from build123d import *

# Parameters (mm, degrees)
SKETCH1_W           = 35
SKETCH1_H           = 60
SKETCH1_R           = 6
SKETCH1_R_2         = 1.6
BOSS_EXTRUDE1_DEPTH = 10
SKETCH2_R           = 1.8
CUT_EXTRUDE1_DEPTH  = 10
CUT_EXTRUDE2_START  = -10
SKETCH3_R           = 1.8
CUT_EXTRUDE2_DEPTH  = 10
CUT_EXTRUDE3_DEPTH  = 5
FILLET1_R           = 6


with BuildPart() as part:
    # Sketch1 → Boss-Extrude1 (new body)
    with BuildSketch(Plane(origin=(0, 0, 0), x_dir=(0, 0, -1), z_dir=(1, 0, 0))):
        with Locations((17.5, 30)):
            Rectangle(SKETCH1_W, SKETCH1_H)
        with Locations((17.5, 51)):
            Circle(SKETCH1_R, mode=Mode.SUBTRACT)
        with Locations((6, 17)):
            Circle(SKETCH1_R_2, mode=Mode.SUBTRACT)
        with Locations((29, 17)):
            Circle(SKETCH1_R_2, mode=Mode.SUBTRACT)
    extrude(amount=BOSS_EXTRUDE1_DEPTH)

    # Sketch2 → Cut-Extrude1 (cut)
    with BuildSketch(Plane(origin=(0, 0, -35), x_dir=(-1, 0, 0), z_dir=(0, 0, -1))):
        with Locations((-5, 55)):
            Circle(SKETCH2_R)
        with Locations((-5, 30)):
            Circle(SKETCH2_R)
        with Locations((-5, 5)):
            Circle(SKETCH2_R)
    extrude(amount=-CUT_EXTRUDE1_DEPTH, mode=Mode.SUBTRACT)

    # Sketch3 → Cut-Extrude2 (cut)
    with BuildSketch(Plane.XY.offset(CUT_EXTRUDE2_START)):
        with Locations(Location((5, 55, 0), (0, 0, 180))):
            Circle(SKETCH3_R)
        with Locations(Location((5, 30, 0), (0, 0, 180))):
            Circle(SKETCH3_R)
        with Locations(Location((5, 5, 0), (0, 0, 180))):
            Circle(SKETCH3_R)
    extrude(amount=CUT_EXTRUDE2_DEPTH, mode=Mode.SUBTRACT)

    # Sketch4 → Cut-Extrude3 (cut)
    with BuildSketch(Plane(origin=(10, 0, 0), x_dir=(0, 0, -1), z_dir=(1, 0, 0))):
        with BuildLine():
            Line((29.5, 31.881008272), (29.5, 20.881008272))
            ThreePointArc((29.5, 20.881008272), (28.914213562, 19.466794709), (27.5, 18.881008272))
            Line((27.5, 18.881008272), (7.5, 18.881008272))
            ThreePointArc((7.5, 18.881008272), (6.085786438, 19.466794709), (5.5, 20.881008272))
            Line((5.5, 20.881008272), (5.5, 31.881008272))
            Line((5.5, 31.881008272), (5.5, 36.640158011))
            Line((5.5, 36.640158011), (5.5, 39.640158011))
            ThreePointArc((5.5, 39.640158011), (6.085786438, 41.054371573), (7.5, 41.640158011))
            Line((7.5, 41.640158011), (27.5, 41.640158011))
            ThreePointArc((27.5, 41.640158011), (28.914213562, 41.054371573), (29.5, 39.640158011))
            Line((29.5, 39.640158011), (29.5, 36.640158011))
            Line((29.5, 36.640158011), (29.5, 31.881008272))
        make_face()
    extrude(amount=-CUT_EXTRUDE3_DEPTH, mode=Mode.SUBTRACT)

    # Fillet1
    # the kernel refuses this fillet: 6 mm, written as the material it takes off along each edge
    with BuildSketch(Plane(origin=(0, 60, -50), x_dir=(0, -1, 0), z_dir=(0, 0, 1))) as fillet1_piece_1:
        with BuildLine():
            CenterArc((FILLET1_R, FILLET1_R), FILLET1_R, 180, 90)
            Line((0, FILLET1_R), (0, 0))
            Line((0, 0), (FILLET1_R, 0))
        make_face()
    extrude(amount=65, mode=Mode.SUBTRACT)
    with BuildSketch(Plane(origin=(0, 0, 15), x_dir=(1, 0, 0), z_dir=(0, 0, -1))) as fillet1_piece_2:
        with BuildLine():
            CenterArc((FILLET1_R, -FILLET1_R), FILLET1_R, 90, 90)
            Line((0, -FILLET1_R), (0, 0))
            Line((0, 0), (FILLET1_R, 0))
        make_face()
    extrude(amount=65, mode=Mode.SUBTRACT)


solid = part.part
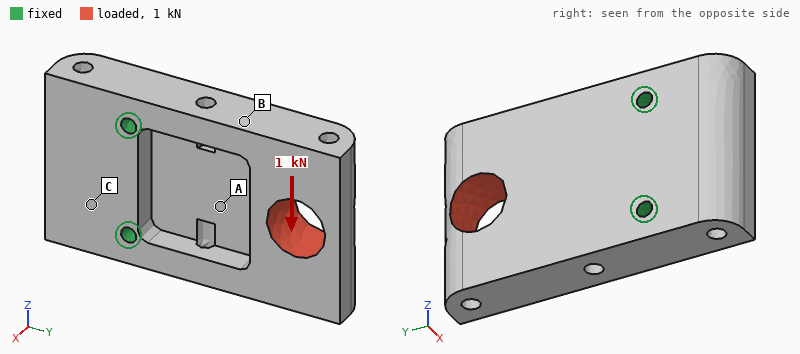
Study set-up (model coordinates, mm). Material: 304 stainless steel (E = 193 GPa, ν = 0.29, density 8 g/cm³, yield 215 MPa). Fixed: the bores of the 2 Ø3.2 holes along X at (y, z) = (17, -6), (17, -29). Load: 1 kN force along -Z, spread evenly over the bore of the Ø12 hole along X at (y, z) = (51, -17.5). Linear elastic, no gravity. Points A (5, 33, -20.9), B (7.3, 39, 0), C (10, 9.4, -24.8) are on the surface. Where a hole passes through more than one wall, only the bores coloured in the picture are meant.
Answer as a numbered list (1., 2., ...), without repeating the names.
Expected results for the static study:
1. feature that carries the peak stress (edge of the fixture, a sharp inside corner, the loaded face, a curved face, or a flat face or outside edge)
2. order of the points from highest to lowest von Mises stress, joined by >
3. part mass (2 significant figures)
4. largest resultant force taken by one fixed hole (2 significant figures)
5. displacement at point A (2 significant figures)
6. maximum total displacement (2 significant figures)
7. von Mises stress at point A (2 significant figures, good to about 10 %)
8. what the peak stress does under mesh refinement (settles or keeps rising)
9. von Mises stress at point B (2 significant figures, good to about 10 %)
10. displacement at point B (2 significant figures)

1. edge of the fixture
2. A > B > C
3. 130 g
4. 1.4 kN
5. 2.8 µm
6. 11 µm
7. 21 MPa
8. keeps rising
9. 7.7 MPa
10. 6.1 µm
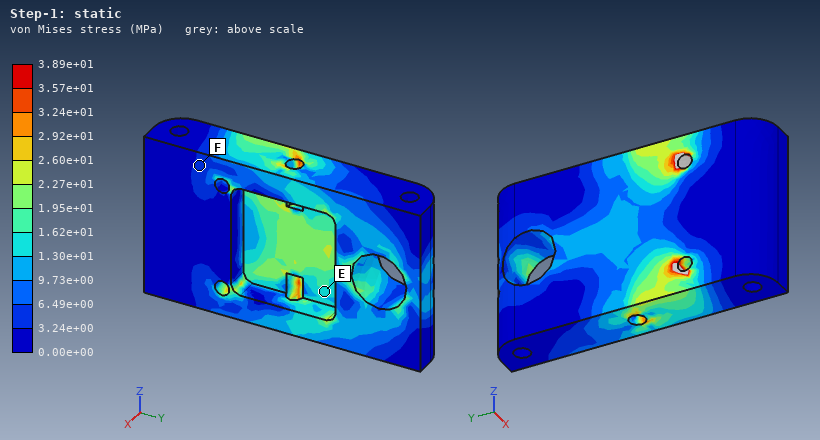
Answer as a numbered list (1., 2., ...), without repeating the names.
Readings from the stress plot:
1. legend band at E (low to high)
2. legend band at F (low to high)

1. 1.30e+01 to 1.62e+01 MPa
2. 3.24e+00 to 6.49e+00 MPa
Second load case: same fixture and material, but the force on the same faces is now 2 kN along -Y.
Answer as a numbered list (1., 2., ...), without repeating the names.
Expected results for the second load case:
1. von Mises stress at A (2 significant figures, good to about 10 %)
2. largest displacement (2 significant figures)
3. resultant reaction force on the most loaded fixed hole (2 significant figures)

1. 16 MPa
2. 11 µm
3. 1.0 kN
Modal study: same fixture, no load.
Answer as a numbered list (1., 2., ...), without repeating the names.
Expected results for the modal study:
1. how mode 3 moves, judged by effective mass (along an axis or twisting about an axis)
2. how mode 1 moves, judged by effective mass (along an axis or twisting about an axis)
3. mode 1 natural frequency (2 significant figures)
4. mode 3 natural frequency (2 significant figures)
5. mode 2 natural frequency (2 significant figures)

1. along Z
2. along X
3. 3300 Hz
4. 10000 Hz
5. 6700 Hz
